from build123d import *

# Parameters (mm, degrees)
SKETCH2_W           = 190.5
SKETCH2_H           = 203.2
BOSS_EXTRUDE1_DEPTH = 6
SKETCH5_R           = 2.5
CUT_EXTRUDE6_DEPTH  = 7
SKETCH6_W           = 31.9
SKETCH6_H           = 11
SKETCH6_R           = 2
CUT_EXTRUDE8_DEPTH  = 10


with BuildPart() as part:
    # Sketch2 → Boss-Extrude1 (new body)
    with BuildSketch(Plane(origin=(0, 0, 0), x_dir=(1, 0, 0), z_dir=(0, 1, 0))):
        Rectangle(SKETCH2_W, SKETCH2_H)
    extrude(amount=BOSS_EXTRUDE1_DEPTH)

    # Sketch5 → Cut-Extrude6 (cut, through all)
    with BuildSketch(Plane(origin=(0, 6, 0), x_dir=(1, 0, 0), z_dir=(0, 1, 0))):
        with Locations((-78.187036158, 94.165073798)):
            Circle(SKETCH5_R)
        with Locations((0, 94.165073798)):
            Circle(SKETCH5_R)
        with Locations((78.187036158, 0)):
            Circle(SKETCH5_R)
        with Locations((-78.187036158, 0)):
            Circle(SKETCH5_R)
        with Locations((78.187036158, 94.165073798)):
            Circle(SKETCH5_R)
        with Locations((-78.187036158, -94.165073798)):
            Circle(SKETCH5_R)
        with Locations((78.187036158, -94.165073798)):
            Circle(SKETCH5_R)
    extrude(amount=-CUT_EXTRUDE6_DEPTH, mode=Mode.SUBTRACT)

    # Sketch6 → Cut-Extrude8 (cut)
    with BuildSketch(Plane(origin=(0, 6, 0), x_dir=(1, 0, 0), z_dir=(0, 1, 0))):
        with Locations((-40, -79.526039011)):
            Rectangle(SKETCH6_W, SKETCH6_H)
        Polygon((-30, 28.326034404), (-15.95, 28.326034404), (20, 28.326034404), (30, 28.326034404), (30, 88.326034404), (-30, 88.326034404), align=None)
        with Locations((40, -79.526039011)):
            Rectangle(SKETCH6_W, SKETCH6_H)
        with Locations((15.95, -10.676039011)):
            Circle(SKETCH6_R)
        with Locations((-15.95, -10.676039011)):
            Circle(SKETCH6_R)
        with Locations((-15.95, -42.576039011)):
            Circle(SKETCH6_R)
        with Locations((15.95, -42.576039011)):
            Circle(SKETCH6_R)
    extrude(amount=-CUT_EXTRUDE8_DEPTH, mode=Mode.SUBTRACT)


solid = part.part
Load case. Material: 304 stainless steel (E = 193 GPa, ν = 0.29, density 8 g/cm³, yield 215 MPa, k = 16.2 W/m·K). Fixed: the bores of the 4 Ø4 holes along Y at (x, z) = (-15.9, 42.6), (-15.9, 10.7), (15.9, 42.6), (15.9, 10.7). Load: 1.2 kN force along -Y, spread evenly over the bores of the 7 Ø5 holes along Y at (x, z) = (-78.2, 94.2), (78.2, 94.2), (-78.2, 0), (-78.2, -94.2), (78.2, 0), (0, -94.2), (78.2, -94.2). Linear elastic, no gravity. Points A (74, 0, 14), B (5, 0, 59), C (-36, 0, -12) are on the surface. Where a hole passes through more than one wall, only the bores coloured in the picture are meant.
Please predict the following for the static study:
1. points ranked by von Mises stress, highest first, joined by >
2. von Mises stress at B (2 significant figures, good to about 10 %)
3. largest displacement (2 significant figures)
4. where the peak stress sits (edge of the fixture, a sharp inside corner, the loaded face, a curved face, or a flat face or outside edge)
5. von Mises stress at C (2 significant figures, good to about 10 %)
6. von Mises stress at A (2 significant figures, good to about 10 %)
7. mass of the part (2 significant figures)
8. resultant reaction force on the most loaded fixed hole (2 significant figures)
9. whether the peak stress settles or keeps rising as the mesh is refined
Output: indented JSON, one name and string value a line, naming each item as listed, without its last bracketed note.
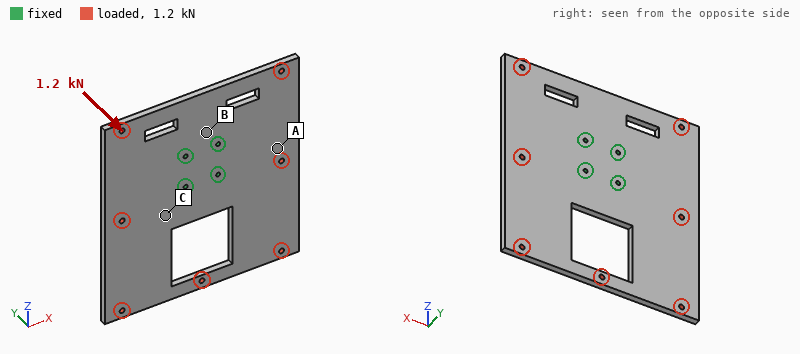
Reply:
{
  "points ranked by von Mises stress, highest first, joined by >": "C > A > B",
  "von Mises stress at B": "8.4 MPa",
  "largest displacement": "0.65 mm",
  "where the peak stress sits": "edge of the fixture",
  "von Mises stress at C": "44 MPa",
  "von Mises stress at A": "30 MPa",
  "mass of the part": "1.6 kg",
  "resultant reaction force on the most loaded fixed hole": "790 N",
  "whether the peak stress settles or keeps rising as the mesh is refined": "keeps rising"
}
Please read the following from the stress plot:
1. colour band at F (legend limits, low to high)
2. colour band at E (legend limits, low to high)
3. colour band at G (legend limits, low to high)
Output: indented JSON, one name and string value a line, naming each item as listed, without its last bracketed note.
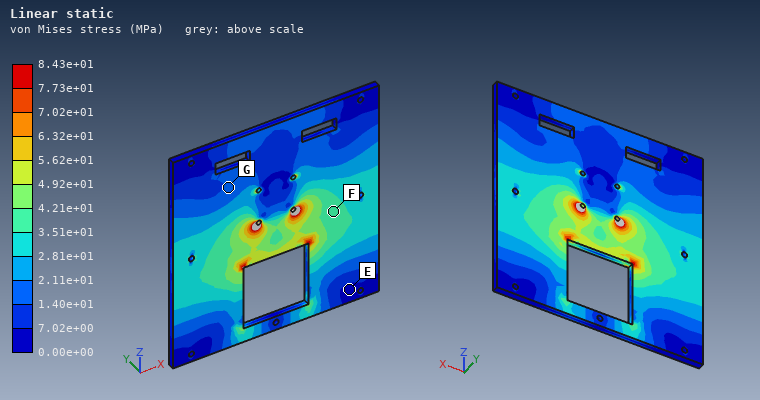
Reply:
{
  "colour band at F": "3.51e+01 to 4.21e+01 MPa",
  "colour band at E": "0.00e+00 to 7.02e+00 MPa",
  "colour band at G": "1.40e+01 to 2.11e+01 MPa"
}
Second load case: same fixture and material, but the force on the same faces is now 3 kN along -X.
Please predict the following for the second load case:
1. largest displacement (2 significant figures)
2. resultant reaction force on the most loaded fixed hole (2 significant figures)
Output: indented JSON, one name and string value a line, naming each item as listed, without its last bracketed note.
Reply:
{
  "largest displacement": "19 µm",
  "resultant reaction force on the most loaded fixed hole": "2.0 kN"
}
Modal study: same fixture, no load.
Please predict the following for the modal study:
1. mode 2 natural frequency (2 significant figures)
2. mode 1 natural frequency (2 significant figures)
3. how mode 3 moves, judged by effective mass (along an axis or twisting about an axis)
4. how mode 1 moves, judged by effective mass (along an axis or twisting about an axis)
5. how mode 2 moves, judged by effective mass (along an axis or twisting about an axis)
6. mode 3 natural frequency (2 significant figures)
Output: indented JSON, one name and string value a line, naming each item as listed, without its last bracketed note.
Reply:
{
  "mode 2 natural frequency": "370 Hz",
  "mode 1 natural frequency": "300 Hz",
  "how mode 3 moves, judged by effective mass": "along Y",
  "how mode 1 moves, judged by effective mass": "along Y",
  "how mode 2 moves, judged by effective mass": "twisting about Z",
  "mode 3 natural frequency": "630 Hz"
}
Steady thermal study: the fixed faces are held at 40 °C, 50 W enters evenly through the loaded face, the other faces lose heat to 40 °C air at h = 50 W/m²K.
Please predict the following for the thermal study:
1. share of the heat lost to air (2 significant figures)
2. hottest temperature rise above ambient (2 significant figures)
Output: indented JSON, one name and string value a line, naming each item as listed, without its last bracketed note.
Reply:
{
  "share of the heat lost to air": "96 %",
  "hottest temperature rise above ambient": "75 K"
}
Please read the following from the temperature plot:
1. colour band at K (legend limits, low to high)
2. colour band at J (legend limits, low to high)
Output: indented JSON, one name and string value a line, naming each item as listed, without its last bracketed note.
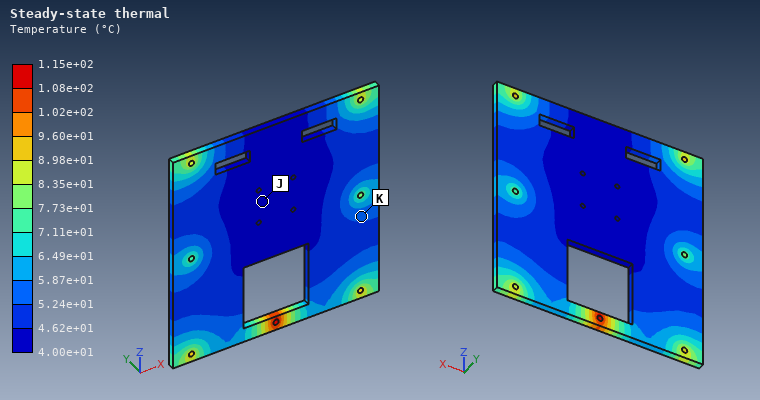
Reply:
{
  "colour band at K": "5.24e+01 to 5.87e+01 °C",
  "colour band at J": "4.00e+01 to 4.62e+01 °C"
}
